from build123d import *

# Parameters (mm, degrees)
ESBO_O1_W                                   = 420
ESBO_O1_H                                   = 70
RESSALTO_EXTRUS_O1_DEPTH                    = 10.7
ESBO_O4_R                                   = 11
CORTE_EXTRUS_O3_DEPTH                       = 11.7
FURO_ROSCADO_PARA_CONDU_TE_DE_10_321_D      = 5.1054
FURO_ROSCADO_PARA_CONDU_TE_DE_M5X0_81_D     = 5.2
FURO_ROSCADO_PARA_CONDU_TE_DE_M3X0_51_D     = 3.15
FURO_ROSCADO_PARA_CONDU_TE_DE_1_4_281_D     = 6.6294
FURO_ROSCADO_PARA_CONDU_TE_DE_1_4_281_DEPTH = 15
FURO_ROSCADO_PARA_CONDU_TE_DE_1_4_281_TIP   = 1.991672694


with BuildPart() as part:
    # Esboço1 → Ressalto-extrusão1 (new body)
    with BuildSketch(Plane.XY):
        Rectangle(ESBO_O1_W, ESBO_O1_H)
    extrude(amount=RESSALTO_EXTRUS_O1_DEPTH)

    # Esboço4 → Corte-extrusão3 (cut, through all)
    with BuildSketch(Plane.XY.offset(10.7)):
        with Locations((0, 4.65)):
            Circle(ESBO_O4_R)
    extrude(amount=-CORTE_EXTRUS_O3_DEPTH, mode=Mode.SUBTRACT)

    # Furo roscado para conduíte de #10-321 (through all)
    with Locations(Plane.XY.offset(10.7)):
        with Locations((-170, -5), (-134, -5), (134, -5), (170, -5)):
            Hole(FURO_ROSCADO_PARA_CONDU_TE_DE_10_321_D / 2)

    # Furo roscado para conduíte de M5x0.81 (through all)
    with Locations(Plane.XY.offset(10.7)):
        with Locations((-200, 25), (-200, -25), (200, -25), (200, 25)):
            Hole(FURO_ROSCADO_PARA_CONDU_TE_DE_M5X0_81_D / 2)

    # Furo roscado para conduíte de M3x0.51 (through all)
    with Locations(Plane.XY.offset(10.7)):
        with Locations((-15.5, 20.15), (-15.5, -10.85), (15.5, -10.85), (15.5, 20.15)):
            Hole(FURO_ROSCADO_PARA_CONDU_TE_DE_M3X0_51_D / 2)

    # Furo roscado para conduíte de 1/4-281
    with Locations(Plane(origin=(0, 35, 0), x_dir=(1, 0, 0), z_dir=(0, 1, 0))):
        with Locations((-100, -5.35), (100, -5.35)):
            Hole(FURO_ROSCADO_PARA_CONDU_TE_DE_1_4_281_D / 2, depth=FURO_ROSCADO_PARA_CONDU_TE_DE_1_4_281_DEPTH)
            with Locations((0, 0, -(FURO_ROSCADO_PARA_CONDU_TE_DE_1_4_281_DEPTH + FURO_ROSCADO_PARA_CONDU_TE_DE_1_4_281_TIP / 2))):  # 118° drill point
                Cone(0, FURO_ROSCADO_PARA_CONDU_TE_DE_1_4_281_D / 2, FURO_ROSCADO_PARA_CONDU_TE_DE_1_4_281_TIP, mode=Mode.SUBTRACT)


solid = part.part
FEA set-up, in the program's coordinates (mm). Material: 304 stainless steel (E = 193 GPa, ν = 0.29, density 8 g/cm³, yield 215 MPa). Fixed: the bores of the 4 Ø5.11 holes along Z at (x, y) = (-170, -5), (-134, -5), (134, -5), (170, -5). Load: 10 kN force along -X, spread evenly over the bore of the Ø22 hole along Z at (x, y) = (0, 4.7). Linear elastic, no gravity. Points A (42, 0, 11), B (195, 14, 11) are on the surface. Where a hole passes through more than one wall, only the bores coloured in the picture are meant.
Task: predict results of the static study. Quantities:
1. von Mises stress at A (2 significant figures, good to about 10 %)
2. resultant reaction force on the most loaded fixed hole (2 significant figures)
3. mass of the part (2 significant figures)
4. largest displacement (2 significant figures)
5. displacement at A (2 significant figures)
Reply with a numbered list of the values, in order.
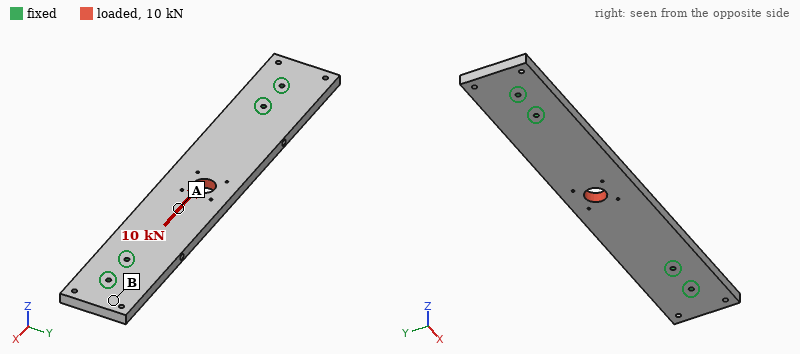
1. 8.6 MPa
2. 3.4 kN
3. 2.5 kg
4. 6.4 µm
5. 4.2 µm
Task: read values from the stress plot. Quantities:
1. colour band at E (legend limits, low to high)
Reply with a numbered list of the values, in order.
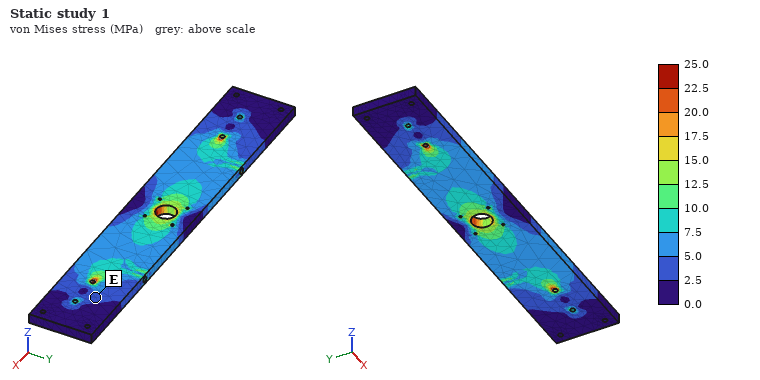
1. 2.5 to 5.0 MPa
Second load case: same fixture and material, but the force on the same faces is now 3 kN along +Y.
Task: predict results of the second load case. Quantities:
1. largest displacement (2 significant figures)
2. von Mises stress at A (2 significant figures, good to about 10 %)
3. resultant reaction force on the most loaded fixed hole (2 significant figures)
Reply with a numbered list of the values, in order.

1. 15 µm
2. 4.9 MPa
3. 3.2 kN
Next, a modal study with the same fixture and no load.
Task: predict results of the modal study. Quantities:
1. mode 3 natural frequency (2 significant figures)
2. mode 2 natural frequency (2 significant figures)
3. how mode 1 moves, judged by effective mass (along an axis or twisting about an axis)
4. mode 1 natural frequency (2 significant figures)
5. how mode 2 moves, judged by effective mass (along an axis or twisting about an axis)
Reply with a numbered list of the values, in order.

1. 1900 Hz
2. 1500 Hz
3. along Z
4. 690 Hz
5. twisting about X
